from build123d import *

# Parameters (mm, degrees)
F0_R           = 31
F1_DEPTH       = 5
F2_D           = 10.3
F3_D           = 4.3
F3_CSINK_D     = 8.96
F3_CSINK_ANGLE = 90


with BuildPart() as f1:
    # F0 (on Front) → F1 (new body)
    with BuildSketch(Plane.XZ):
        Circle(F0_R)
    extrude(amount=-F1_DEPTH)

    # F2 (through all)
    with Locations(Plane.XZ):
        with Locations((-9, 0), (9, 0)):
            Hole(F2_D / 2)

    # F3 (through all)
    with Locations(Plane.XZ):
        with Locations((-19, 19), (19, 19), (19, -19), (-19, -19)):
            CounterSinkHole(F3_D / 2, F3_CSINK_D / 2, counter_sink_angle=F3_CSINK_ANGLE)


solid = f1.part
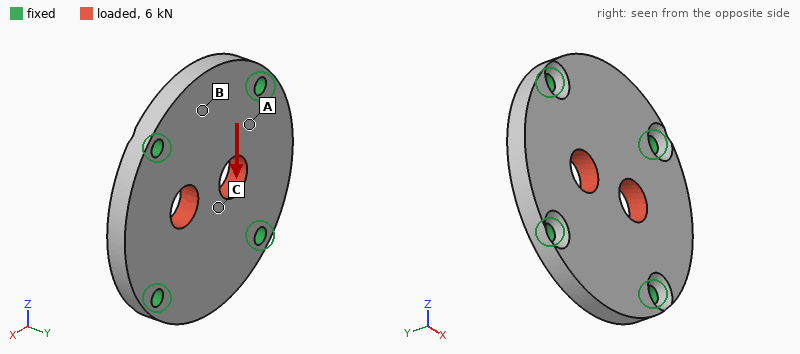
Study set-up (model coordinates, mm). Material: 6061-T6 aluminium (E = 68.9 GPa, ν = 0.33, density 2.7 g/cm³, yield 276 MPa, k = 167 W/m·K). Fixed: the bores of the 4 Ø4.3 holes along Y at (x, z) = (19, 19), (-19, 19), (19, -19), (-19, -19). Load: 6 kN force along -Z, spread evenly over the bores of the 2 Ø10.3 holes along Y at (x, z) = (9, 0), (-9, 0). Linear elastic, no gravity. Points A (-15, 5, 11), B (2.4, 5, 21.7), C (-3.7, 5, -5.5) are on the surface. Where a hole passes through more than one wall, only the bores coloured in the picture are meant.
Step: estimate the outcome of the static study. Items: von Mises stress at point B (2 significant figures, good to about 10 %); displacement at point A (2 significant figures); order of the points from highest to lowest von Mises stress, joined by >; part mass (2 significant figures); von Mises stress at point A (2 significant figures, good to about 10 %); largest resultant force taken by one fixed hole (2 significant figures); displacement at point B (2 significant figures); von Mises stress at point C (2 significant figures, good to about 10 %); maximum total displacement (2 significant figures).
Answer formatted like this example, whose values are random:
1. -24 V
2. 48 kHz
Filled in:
1. 8.1 MPa
2. 4.1 µm
3. A > C > B
4. 37 g
5. 27 MPa
6. 1.5 kN
7. 6.3 µm
8. 16 MPa
9. 10 µm
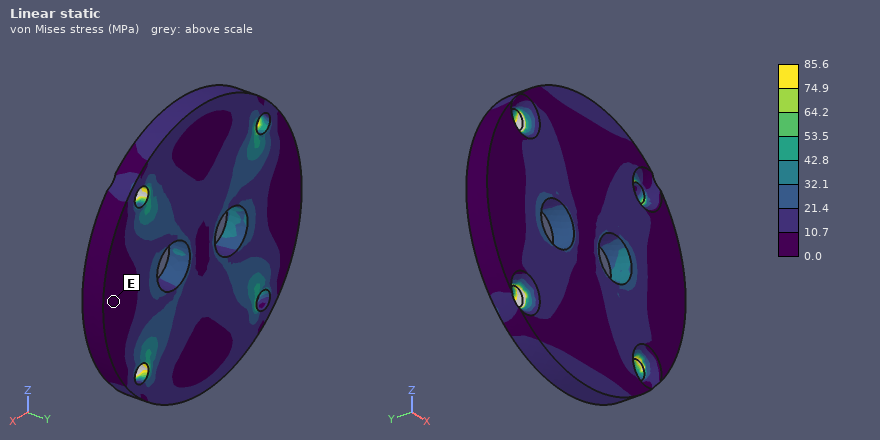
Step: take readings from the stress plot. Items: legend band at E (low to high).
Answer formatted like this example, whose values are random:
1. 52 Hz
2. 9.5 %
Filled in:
1. 0.0 to 10.7 MPa
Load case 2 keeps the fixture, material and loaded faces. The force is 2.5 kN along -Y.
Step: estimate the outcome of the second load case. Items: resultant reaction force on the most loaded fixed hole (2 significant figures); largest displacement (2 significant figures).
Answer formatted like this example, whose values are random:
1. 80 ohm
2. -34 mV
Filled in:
1. 900 N
2. 80 µm
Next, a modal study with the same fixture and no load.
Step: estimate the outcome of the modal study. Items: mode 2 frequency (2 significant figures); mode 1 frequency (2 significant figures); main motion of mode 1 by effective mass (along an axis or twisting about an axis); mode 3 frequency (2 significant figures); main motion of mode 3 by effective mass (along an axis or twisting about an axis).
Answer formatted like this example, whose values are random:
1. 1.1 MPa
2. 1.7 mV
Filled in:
1. 11 kHz
2. 11 kHz
3. along Y
4. 12 kHz
5. twisting about X
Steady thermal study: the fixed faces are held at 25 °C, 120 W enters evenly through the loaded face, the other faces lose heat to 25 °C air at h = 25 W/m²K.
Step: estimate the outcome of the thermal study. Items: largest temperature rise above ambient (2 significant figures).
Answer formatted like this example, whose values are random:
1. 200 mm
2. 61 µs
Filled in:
1. 44 K
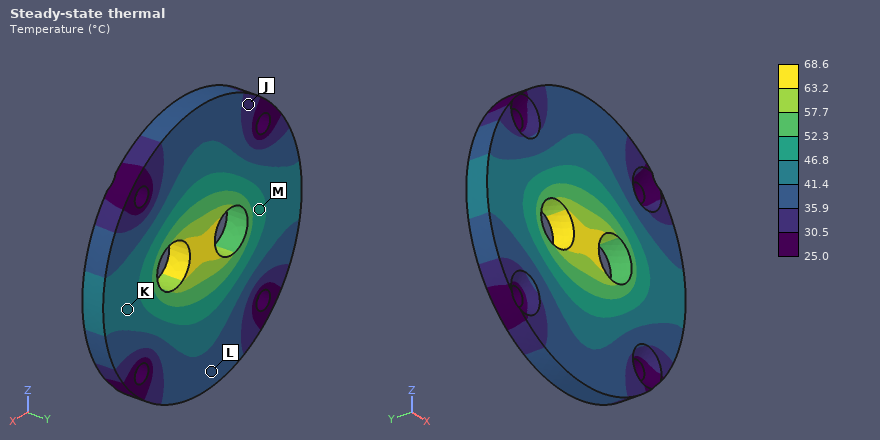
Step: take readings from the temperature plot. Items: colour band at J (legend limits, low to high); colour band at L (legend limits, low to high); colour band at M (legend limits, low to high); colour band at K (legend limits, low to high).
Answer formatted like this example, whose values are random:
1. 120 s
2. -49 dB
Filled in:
1. 30.5 to 35.9 °C
2. 35.9 to 41.4 °C
3. 46.8 to 52.3 °C
4. 41.4 to 46.8 °C
